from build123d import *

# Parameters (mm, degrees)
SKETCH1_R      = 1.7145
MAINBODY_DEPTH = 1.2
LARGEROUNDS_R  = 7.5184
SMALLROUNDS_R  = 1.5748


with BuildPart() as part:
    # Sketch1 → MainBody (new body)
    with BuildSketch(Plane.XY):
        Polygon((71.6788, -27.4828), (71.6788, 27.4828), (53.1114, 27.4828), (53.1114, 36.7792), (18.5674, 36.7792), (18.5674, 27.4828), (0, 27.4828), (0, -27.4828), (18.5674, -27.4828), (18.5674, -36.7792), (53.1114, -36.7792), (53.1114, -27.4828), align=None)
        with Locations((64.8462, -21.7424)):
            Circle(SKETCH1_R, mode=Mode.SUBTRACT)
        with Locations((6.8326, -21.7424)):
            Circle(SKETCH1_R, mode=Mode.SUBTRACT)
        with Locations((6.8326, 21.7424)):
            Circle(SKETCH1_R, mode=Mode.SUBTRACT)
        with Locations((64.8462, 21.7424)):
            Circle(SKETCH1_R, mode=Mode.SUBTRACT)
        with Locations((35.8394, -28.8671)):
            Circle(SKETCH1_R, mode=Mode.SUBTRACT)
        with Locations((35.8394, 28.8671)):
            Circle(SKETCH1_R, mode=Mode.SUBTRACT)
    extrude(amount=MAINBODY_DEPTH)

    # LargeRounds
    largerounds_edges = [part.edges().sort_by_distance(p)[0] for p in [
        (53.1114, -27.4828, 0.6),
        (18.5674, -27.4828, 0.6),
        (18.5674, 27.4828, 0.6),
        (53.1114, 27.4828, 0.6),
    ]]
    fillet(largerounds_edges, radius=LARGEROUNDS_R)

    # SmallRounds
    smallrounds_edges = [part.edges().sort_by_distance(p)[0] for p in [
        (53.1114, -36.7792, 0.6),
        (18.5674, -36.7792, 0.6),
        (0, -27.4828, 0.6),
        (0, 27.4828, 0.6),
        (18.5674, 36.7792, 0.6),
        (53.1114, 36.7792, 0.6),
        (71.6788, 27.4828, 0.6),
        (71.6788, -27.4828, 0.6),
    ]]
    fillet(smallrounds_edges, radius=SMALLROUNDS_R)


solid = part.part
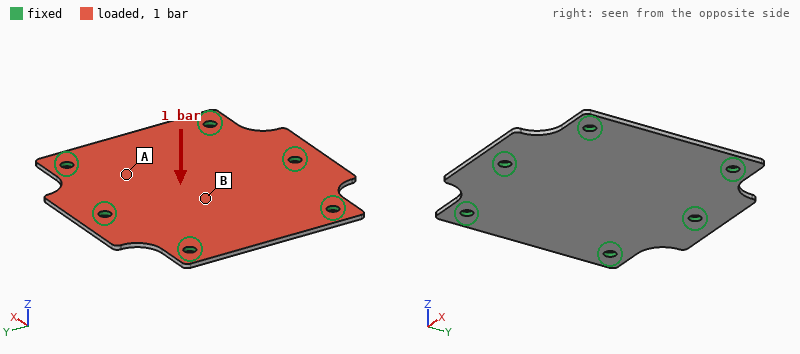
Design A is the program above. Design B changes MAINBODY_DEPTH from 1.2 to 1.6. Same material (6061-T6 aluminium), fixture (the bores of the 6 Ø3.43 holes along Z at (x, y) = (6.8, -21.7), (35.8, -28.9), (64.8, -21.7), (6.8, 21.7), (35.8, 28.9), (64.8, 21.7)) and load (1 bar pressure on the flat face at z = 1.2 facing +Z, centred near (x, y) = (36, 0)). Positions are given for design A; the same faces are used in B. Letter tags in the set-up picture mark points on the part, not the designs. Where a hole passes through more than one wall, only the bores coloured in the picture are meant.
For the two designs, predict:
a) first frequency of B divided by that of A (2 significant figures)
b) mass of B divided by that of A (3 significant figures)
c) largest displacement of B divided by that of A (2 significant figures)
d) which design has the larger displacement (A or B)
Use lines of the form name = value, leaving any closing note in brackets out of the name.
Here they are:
first frequency of B divided by that of A = 1.3
mass of B divided by that of A = 1.33
largest displacement of B divided by that of A = 0.43
which design has the larger displacement = A
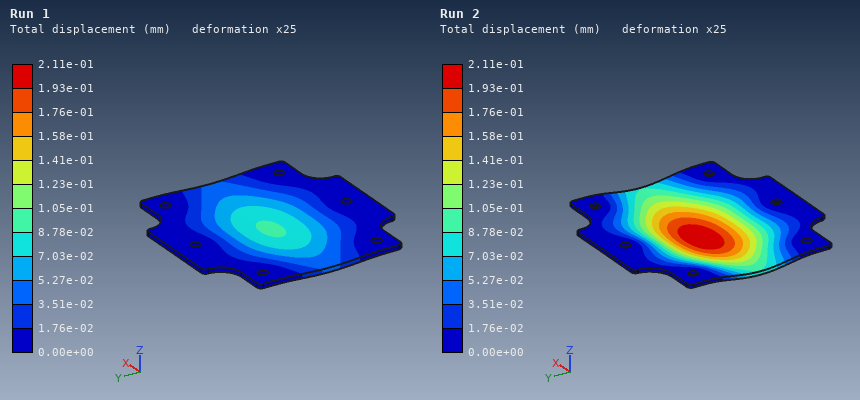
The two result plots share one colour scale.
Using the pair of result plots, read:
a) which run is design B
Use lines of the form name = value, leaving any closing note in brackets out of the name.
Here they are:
which run is design B = Run 1
